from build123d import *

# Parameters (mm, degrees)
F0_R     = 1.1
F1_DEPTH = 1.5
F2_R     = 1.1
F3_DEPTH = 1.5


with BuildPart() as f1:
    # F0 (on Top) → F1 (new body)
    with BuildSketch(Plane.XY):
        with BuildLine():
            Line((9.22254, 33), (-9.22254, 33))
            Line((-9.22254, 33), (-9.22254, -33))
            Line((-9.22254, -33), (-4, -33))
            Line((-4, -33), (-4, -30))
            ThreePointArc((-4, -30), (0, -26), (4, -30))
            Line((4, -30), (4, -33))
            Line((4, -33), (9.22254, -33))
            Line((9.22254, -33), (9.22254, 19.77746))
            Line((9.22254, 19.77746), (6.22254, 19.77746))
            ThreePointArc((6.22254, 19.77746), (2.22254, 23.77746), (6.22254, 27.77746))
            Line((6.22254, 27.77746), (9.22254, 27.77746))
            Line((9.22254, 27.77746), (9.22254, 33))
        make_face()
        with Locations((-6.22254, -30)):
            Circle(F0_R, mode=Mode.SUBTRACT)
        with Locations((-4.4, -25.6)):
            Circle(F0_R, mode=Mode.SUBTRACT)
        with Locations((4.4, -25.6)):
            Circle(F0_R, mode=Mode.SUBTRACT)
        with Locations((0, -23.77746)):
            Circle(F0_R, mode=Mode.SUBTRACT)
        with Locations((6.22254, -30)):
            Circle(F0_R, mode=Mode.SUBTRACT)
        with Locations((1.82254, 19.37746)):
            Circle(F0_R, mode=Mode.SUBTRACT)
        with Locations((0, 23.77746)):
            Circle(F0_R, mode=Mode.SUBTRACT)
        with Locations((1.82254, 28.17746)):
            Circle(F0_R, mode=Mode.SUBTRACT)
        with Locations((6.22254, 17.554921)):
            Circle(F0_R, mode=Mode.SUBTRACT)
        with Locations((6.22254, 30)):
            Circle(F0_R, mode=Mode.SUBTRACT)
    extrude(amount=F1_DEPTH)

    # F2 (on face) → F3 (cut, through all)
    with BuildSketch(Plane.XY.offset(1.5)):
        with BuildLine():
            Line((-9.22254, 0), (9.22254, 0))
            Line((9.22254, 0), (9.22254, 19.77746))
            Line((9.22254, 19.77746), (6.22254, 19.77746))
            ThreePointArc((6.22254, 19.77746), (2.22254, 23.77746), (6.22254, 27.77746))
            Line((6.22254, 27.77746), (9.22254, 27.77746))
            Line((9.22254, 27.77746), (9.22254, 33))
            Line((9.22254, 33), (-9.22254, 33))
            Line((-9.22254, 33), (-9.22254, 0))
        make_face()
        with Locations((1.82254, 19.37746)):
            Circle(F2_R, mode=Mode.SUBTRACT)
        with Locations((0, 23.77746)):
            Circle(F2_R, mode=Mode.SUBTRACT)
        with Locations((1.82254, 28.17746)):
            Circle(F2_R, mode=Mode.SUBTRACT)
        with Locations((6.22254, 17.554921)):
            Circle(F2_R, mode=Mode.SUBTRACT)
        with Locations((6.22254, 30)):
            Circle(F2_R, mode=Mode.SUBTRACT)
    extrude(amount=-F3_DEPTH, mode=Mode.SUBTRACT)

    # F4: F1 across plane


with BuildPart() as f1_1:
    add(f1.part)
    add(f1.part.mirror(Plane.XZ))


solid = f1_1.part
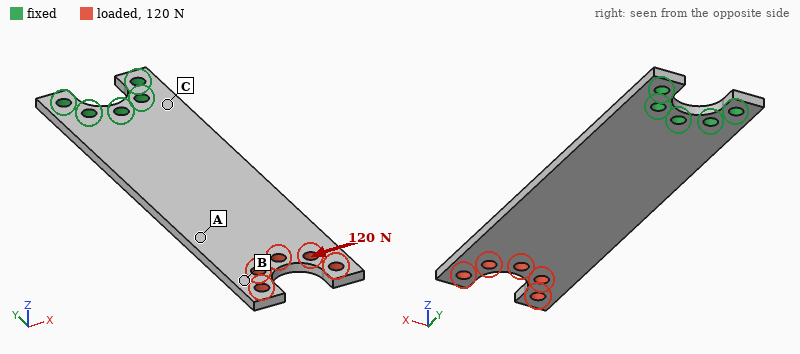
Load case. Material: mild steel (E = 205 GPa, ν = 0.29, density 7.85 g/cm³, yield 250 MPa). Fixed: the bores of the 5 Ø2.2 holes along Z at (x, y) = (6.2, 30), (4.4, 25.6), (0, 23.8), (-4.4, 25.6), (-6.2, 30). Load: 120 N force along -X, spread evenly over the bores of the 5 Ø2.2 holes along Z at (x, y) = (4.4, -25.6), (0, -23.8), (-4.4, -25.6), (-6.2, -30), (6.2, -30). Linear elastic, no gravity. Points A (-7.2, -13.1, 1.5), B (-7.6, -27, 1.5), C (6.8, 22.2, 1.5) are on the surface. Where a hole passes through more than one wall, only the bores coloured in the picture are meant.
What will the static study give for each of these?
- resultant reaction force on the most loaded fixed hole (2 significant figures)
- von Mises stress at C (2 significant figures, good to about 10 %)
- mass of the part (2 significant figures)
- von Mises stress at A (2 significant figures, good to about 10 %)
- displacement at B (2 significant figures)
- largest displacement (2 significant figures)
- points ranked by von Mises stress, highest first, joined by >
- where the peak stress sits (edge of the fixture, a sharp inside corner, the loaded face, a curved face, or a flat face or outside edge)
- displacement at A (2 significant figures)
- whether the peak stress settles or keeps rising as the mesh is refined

350 N
51 MPa
13 g
16 MPa
44 µm
51 µm
C > A > B
edge of the fixture
28 µm
keeps rising
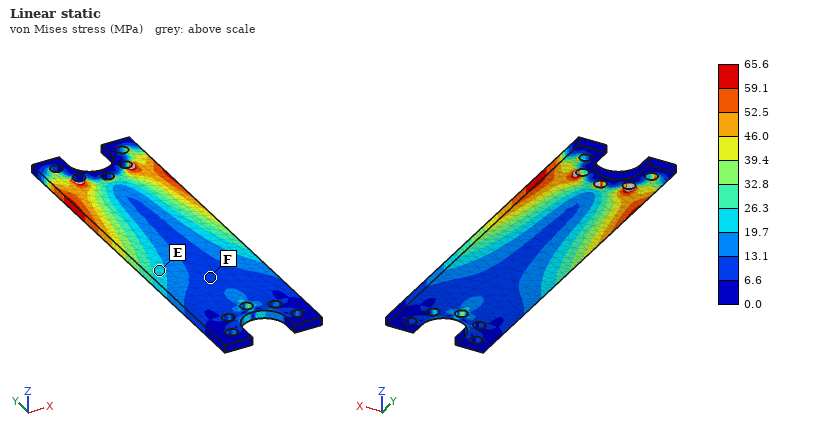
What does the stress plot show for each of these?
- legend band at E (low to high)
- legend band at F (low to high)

19.7 to 26.3 MPa
6.6 to 13.1 MPa
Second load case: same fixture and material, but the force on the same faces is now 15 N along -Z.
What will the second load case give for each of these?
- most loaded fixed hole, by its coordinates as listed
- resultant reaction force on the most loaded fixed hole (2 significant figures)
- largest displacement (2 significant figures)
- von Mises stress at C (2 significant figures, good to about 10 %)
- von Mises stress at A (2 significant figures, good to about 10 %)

(0, 23.8)
81 N
0.71 mm
77 MPa
30 MPa
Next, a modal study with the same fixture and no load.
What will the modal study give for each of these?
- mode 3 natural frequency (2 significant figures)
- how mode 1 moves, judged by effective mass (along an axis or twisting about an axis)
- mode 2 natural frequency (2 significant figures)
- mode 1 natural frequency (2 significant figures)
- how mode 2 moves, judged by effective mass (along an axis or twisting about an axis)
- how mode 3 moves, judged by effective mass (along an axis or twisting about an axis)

2600 Hz
along Z
2400 Hz
440 Hz
twisting about Y
along Z
